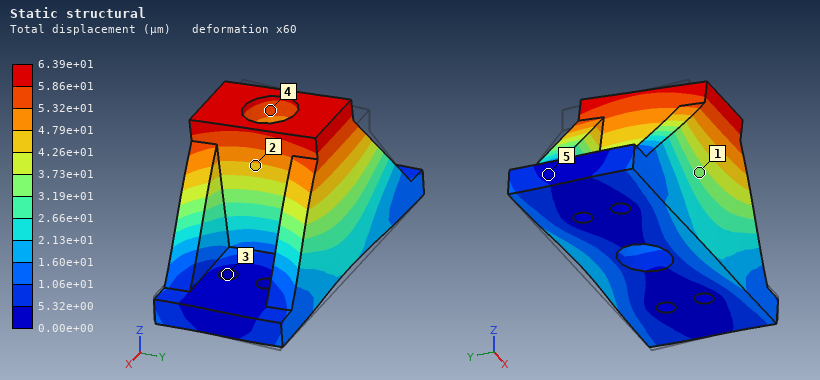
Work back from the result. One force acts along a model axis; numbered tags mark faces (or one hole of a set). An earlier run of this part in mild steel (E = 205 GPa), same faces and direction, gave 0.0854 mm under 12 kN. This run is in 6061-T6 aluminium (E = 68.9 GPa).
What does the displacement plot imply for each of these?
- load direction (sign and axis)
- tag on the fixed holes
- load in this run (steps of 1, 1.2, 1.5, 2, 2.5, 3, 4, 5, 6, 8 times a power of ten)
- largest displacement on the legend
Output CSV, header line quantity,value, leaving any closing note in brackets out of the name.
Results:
quantity,value
load direction,-Y
tag on the fixed holes,3
load in this run,3 kN
largest displacement on the legend,6.39e+01 µm
